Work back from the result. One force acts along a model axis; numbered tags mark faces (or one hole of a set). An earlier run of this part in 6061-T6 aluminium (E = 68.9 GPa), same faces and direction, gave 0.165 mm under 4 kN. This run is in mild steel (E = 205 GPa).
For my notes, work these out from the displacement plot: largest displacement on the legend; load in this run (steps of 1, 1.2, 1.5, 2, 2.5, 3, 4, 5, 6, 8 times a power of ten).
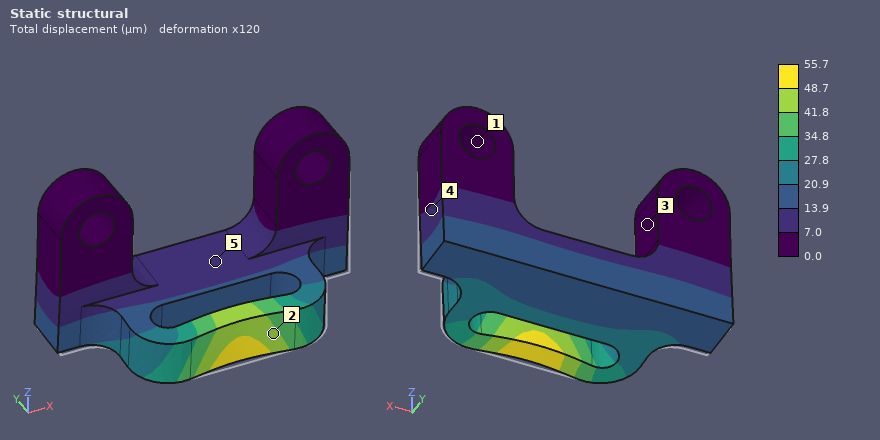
55.7 µm
4 kN
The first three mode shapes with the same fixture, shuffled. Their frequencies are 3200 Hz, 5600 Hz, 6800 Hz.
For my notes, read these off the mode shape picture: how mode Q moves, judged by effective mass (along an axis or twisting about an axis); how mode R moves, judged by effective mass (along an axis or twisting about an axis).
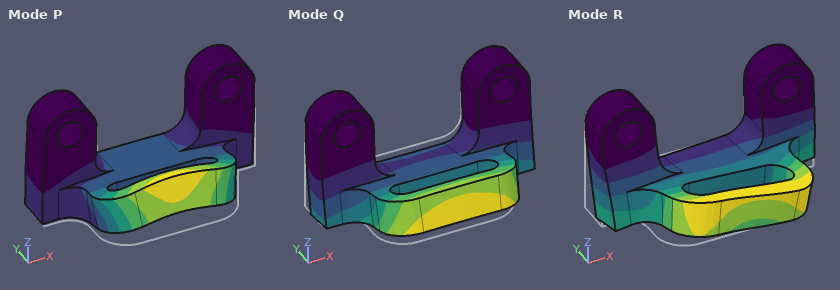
along Y
along X
